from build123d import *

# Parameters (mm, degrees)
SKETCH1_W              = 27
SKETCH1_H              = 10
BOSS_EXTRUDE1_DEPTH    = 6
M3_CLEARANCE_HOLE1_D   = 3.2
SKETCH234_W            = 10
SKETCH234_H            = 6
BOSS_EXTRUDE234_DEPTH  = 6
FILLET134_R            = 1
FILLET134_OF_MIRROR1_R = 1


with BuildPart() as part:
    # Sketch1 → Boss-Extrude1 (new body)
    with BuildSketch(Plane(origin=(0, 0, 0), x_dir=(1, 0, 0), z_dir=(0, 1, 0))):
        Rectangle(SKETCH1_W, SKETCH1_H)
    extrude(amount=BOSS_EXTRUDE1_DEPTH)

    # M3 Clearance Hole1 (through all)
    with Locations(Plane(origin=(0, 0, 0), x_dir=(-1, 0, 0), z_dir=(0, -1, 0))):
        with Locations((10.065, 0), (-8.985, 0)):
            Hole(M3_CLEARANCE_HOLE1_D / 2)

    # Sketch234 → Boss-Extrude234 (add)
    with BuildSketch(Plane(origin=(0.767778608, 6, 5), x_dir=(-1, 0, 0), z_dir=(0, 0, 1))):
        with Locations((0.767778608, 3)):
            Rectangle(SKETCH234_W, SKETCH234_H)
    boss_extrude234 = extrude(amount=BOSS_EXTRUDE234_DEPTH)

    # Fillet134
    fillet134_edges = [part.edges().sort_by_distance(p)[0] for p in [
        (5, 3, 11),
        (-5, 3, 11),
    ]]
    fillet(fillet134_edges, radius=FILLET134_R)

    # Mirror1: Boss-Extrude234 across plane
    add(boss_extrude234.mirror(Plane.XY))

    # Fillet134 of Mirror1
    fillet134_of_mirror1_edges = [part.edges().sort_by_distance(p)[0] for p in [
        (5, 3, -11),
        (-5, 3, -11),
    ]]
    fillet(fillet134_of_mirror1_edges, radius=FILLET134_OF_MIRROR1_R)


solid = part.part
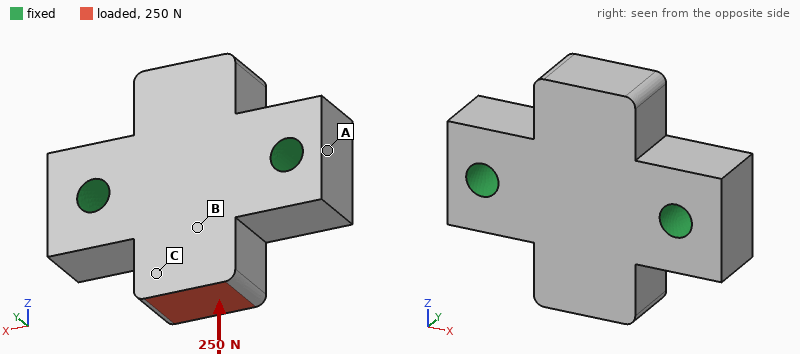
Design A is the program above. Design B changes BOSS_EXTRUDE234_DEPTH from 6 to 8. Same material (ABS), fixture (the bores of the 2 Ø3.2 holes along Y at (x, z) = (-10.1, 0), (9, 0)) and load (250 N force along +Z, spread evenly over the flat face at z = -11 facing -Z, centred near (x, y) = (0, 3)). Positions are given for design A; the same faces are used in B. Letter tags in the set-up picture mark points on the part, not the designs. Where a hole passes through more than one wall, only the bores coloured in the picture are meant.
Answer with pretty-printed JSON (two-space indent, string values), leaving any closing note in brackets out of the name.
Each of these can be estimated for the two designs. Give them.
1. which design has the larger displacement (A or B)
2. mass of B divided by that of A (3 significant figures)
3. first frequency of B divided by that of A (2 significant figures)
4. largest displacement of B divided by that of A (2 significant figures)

{
  "which design has the larger displacement": "B",
  "mass of B divided by that of A": "1.11",
  "first frequency of B divided by that of A": "0.77",
  "largest displacement of B divided by that of A": "1.1"
}
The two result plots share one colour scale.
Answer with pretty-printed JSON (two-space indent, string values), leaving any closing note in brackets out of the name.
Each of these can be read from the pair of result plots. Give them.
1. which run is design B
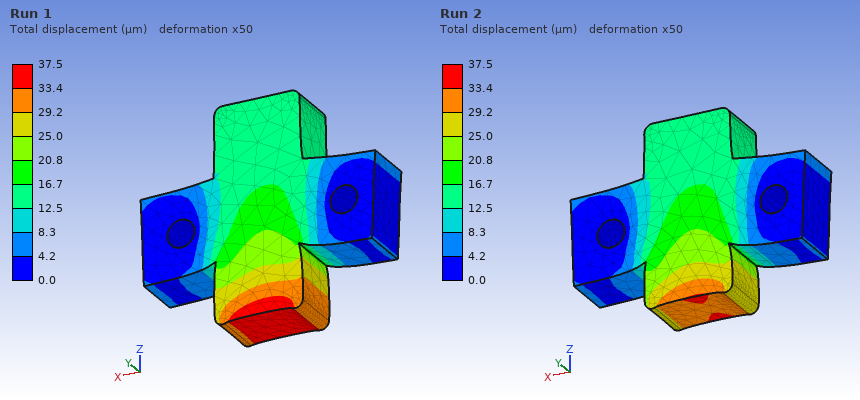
{
  "which run is design B": "Run 1"
}
